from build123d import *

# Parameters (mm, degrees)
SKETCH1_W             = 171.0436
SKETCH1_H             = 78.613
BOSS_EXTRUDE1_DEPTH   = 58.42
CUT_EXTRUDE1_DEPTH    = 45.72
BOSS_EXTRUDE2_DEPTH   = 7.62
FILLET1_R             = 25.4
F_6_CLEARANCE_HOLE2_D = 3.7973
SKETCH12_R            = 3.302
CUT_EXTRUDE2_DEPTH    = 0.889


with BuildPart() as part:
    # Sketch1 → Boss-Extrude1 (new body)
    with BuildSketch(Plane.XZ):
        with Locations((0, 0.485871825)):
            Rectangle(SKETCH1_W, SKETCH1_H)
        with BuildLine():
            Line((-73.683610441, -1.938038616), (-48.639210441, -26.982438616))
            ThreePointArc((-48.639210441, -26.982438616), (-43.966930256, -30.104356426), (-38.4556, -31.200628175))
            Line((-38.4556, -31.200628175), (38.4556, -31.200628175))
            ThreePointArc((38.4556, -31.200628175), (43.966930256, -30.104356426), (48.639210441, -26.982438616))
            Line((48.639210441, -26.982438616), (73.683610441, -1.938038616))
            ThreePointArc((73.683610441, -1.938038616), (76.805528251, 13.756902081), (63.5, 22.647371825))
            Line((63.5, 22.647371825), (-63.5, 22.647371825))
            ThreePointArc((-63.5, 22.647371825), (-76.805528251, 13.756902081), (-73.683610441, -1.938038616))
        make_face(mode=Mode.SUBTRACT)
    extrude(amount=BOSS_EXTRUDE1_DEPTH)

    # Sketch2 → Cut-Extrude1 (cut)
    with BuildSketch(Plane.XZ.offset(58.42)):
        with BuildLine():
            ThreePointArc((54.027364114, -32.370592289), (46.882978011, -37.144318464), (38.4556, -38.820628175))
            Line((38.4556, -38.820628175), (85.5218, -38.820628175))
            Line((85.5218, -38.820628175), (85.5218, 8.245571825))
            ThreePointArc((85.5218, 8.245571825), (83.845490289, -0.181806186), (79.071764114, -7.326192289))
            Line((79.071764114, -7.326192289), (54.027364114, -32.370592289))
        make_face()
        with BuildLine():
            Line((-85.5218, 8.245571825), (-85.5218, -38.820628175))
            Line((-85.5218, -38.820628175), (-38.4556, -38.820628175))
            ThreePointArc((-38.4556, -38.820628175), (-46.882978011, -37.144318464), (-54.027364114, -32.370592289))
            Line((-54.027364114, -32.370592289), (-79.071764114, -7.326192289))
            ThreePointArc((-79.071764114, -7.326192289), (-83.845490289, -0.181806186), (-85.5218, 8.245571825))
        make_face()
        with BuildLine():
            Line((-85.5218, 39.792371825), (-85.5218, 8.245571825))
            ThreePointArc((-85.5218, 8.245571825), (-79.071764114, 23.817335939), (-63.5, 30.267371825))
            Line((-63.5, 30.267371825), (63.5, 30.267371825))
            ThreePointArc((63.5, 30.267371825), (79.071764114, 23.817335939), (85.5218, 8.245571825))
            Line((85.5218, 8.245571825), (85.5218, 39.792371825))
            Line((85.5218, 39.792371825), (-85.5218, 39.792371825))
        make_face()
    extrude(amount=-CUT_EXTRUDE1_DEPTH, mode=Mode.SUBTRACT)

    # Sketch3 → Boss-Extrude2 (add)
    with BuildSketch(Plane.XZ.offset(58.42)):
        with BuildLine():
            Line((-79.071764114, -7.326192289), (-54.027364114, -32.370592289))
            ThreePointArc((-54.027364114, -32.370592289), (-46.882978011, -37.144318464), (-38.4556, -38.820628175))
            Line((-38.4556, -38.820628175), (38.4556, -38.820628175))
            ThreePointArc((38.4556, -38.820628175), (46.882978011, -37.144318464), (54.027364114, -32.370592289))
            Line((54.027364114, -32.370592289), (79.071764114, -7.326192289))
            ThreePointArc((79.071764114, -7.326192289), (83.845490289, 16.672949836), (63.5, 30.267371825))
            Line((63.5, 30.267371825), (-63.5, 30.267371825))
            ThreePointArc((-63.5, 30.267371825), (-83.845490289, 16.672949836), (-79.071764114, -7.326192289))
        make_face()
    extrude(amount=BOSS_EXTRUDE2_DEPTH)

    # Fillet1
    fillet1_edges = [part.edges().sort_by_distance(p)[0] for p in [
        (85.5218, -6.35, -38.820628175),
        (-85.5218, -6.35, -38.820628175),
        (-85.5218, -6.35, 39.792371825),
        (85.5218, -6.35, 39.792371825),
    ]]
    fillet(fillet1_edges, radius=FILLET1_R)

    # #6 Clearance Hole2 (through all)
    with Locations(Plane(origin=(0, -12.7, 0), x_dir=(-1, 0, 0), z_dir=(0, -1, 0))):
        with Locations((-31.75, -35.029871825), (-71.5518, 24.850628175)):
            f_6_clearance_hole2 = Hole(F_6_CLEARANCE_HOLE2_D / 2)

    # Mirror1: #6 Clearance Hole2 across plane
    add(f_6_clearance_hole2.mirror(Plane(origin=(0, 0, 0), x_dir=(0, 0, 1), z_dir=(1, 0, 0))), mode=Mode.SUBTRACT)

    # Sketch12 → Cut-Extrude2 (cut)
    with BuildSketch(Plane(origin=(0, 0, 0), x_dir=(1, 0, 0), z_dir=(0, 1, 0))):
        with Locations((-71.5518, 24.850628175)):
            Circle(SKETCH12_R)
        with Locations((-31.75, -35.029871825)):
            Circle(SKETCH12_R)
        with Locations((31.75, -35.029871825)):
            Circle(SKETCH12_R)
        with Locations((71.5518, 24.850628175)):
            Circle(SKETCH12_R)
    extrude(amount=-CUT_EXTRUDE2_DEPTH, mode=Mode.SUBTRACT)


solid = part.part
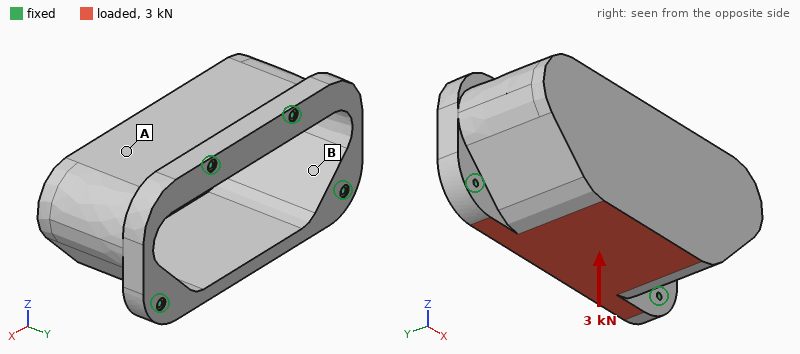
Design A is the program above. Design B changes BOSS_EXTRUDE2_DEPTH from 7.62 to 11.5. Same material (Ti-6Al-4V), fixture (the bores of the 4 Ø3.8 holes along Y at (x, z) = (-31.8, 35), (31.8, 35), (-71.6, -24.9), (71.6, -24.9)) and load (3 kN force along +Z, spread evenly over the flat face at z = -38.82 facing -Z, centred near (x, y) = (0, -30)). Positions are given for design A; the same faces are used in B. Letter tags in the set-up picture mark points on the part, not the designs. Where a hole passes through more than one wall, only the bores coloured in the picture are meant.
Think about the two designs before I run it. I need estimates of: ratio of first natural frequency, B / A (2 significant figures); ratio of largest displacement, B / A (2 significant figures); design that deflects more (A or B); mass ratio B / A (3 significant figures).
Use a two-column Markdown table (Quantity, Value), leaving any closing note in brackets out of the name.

| Quantity | Value |
|---|---|
| ratio of first natural frequency, B / A | 0.90 |
| ratio of largest displacement, B / A | 0.92 |
| design that deflects more | A |
| mass ratio B / A | 1.14 |
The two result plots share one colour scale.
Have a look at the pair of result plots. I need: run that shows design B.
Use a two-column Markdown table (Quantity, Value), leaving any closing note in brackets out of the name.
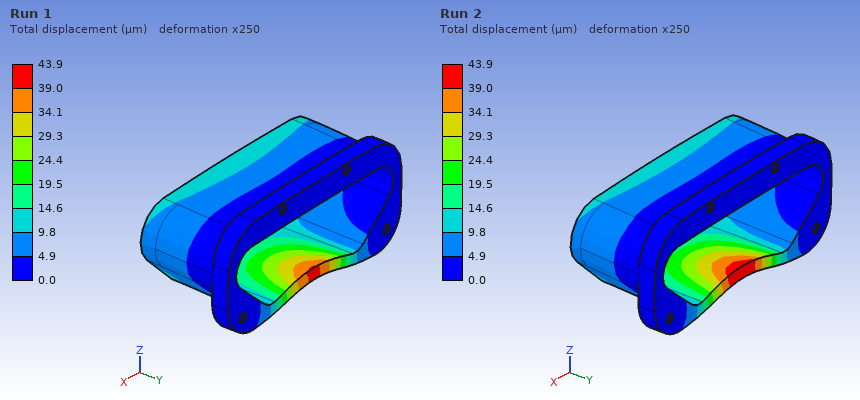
| Quantity | Value |
|---|---|
| run that shows design B | Run 1 |
